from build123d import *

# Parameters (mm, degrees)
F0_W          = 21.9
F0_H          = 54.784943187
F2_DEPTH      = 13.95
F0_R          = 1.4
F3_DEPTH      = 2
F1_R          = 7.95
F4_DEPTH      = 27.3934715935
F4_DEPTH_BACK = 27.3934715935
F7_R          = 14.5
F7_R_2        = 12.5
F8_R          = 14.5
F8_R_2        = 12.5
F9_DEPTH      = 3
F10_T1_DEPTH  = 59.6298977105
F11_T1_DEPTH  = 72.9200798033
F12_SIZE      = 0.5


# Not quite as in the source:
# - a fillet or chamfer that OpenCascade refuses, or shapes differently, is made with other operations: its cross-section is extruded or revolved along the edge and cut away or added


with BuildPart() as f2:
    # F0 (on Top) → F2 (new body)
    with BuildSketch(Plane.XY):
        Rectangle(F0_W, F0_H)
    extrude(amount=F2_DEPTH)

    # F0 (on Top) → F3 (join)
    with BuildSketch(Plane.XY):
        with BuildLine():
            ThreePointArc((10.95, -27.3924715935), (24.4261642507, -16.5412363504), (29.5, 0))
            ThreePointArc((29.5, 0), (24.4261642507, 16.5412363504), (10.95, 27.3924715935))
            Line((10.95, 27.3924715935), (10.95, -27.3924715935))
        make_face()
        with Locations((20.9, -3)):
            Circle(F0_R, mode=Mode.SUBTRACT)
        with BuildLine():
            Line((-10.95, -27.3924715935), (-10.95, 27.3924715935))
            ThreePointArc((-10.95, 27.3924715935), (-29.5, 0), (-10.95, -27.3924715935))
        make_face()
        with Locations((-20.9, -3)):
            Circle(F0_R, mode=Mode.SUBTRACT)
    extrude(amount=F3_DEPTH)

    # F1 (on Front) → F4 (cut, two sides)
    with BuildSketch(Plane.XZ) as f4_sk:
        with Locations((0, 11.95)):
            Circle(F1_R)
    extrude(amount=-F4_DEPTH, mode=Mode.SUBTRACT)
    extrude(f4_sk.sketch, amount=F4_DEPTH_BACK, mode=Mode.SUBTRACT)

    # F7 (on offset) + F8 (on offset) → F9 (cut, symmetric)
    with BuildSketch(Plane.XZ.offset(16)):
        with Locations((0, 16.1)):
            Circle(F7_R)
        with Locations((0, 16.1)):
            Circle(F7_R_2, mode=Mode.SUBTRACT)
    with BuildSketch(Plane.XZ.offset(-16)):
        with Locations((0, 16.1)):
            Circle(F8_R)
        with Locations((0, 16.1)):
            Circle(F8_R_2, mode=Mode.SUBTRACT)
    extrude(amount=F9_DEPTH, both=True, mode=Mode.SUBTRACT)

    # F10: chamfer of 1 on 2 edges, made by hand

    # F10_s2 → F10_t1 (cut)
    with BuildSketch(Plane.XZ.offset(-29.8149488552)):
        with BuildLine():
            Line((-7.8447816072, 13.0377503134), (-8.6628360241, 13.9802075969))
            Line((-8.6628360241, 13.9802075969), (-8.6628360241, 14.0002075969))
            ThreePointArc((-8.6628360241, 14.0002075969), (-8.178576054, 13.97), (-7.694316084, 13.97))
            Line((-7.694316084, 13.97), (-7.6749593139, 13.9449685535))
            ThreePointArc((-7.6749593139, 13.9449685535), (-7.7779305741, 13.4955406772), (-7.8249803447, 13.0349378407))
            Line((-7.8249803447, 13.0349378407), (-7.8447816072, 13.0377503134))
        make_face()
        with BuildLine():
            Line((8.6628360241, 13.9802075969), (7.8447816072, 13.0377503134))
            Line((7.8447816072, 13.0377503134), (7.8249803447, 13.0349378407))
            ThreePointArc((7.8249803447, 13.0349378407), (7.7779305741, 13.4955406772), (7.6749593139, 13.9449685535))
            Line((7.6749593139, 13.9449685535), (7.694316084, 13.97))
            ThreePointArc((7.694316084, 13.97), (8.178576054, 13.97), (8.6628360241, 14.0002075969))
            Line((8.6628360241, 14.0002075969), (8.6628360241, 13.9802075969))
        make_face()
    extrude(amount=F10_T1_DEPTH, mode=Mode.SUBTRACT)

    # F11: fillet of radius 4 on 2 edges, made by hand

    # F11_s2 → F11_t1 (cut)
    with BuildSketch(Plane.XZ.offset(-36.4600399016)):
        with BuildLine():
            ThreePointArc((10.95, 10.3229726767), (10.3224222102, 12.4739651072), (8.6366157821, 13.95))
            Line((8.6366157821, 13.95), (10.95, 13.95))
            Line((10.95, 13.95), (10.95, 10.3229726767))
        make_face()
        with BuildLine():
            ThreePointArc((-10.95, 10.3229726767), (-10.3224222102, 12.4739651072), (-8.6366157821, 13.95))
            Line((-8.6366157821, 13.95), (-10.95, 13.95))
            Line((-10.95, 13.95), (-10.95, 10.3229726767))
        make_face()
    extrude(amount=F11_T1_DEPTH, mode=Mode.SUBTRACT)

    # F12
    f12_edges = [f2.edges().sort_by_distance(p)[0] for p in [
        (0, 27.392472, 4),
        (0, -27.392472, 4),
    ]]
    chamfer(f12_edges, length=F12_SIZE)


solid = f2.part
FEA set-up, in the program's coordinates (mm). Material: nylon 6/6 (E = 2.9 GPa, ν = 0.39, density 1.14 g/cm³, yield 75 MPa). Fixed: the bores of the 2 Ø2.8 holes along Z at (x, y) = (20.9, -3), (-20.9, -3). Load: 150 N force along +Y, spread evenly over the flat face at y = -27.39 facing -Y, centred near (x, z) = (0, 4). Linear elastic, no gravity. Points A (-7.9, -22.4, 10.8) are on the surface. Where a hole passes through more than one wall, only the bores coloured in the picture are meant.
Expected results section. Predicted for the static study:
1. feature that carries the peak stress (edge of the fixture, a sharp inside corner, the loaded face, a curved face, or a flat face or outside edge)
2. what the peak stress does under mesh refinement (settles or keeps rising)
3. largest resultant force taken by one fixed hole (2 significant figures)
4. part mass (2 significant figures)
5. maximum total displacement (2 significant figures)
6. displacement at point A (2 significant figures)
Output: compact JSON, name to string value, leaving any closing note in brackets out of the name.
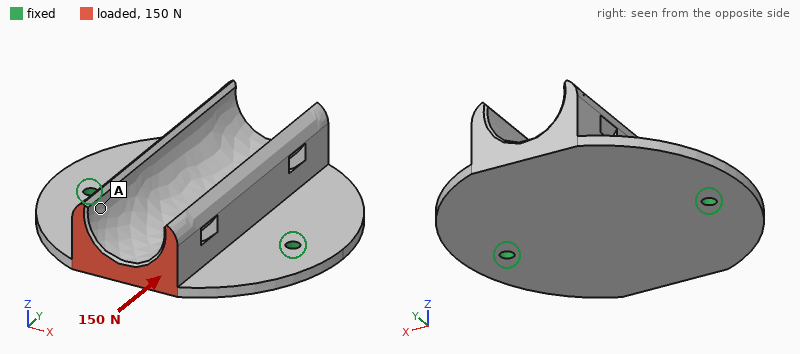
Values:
{"feature that carries the peak stress": "edge of the fixture", "what the peak stress does under mesh refinement": "keeps rising", "largest resultant force taken by one fixed hole": "75 N", "part mass": "13 g", "maximum total displacement": "0.81 mm", "displacement at point A": "0.54 mm"}
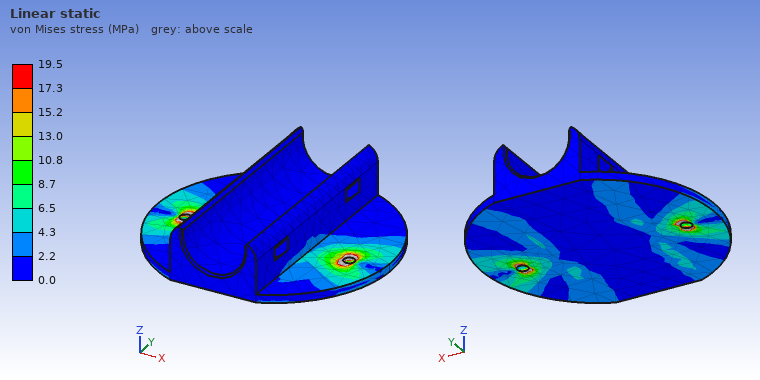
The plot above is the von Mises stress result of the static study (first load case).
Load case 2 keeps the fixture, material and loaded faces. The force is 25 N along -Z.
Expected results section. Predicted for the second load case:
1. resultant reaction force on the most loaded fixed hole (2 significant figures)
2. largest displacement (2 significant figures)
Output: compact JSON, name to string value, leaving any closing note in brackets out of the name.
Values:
{"resultant reaction force on the most loaded fixed hole": "18 N", "largest displacement": "0.88 mm"}
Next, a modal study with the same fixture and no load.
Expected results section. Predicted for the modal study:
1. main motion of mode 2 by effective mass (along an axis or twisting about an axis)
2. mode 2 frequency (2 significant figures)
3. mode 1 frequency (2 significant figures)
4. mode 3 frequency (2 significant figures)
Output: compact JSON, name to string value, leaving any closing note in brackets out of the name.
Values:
{"main motion of mode 2 by effective mass": "along Z", "mode 2 frequency": "1100 Hz", "mode 1 frequency": "410 Hz", "mode 3 frequency": "1800 Hz"}
